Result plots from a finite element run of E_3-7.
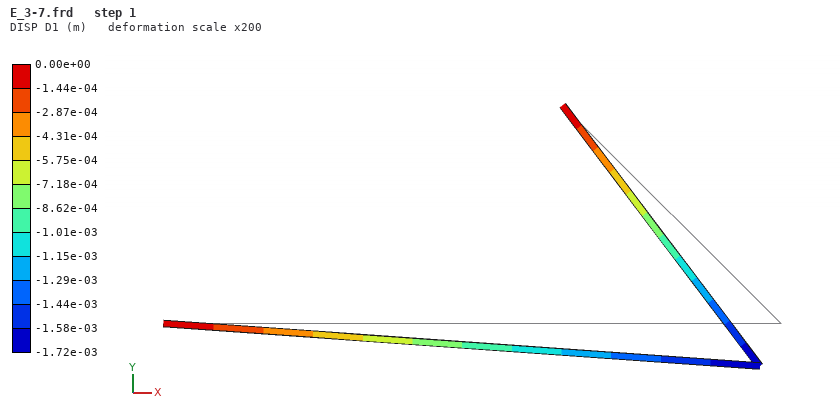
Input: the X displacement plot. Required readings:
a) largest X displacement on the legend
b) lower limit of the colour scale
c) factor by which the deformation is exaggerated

0.00e+00 m
-1.72e-03 m
200
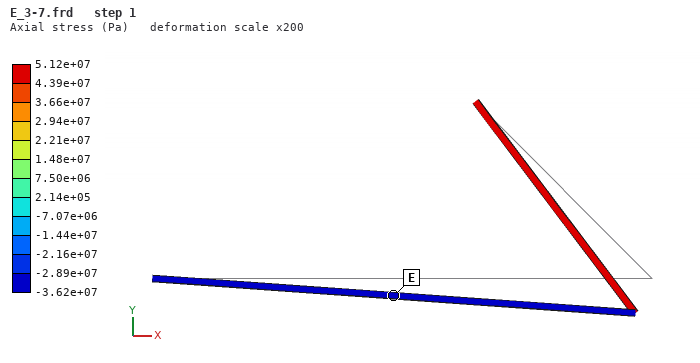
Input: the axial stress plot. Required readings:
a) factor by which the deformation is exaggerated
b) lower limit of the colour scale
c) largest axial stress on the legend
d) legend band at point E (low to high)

200
-3.62e+07 Pa
5.12e+07 Pa
-3.62e+07 to -2.89e+07 Pa
